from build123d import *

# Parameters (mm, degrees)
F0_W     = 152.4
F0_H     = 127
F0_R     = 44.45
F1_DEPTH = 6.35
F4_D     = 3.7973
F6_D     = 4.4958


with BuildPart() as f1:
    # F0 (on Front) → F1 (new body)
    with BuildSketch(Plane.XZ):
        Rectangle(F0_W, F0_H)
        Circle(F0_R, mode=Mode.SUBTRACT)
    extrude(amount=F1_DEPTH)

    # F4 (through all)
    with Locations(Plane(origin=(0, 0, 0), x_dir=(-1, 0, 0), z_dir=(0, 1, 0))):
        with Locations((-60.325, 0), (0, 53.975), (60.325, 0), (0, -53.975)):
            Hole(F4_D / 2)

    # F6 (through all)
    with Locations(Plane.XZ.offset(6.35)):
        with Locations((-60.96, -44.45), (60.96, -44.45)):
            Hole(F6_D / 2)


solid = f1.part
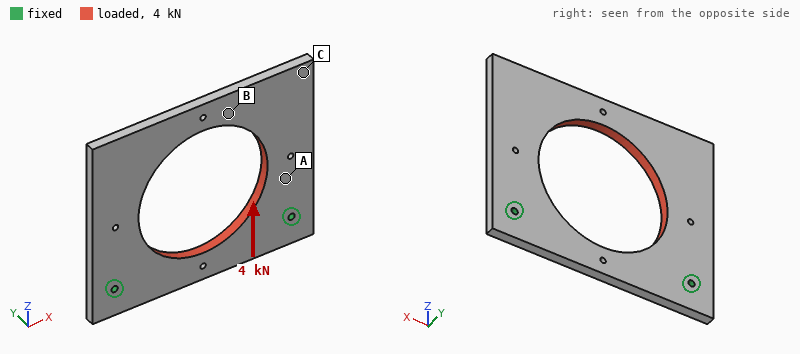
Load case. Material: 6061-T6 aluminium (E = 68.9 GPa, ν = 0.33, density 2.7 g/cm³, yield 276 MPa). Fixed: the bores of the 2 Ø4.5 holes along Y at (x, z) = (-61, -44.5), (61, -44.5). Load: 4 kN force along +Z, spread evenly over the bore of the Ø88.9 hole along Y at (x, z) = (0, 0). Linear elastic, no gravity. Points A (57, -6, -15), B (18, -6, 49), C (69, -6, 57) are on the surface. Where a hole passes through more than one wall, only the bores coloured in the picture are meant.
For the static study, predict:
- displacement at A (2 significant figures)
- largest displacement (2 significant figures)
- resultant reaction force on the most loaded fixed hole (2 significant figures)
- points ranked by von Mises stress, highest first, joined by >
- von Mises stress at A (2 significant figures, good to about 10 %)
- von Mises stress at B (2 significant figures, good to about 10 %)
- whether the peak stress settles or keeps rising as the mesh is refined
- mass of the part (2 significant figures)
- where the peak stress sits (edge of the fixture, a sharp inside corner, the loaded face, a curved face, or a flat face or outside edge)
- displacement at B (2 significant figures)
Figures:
5.6 µm
17 µm
2.0 kN
A > B > C
9.0 MPa
5.1 MPa
keeps rising
220 g
edge of the fixture
15 µm
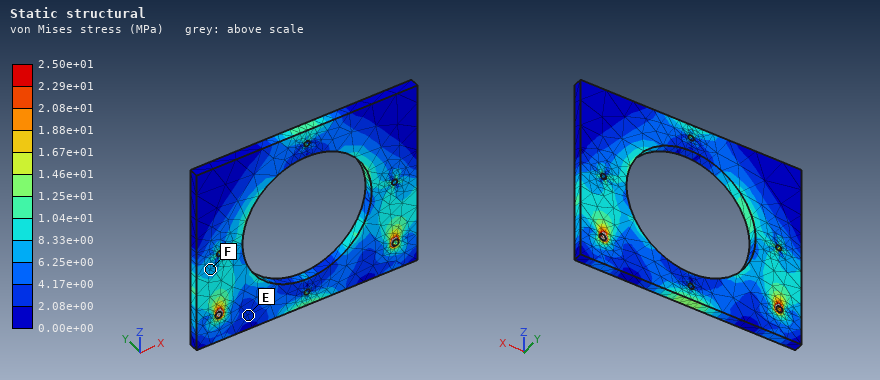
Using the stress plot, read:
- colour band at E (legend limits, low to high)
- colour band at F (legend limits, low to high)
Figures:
2.08e+00 to 4.17e+00 MPa
6.25e+00 to 8.33e+00 MPa
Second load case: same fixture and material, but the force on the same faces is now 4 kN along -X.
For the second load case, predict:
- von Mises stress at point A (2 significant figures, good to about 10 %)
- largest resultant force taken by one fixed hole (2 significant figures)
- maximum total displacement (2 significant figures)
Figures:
14 MPa
2.4 kN
94 µm
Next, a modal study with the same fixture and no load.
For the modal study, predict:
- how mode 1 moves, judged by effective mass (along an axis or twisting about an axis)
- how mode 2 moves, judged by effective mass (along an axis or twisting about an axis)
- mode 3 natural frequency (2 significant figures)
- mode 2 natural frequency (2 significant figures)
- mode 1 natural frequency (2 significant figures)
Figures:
along Y
twisting about Z
1600 Hz
670 Hz
320 Hz
